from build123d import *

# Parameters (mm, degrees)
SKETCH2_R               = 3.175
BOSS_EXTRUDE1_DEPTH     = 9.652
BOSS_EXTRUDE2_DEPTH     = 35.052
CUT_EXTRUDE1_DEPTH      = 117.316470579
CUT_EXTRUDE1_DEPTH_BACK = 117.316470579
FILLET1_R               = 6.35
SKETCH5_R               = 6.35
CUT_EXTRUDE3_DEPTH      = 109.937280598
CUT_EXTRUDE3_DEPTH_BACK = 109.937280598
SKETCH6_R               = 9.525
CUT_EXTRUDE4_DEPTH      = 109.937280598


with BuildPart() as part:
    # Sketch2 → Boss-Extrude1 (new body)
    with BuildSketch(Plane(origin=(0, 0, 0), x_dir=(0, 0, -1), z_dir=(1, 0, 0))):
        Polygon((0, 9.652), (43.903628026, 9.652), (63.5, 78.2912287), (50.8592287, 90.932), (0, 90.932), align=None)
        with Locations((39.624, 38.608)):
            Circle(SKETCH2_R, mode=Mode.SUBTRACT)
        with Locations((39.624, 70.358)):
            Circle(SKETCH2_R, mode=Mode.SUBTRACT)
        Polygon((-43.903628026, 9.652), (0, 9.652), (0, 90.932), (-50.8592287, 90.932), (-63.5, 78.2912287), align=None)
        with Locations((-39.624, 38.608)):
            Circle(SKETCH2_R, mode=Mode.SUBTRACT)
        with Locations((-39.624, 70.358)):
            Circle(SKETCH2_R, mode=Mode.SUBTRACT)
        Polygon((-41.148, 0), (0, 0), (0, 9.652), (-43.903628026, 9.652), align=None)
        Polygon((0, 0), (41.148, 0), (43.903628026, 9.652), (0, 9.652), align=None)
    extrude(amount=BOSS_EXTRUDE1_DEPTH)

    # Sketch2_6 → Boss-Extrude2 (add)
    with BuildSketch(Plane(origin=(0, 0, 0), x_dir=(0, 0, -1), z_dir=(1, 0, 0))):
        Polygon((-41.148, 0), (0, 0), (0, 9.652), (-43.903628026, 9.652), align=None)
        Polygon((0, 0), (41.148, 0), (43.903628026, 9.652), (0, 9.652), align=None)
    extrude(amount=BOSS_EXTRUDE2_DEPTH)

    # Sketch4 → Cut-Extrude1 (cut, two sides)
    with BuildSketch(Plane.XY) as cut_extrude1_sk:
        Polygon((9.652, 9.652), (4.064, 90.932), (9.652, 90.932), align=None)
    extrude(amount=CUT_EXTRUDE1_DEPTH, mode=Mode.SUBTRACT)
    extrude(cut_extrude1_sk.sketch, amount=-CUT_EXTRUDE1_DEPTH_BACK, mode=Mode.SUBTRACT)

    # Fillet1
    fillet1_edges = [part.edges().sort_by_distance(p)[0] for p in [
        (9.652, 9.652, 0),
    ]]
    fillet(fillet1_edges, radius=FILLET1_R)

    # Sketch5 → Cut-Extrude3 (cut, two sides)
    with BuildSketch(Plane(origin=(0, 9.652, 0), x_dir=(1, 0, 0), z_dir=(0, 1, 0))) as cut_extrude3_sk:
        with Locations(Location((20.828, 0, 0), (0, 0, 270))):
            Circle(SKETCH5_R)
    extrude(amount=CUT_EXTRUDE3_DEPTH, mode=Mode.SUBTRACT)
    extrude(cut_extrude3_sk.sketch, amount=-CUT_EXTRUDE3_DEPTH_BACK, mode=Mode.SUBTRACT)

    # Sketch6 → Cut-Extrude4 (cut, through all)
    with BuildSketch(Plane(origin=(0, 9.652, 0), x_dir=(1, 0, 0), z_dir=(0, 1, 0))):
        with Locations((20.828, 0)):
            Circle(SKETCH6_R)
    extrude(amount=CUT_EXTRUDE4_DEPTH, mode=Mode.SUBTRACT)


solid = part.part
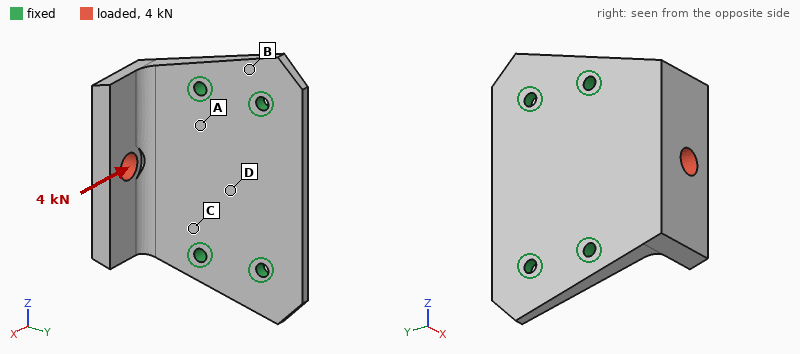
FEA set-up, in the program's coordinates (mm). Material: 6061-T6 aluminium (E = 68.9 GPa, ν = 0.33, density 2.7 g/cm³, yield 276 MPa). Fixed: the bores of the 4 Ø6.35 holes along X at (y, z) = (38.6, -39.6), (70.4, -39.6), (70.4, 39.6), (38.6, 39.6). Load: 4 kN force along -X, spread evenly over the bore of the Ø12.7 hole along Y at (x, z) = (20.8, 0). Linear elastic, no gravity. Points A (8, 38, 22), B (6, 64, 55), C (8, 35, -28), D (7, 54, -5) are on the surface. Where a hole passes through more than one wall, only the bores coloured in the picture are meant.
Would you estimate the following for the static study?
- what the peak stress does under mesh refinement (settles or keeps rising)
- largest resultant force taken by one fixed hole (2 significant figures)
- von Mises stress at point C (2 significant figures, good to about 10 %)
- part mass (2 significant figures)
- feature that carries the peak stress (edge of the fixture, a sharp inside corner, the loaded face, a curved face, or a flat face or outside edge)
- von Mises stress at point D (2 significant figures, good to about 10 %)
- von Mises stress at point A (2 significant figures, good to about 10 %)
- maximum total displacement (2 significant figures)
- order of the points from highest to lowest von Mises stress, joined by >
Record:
keeps rising
2.7 kN
85 MPa
230 g
edge of the fixture
30 MPa
67 MPa
0.40 mm
C > A > D > B
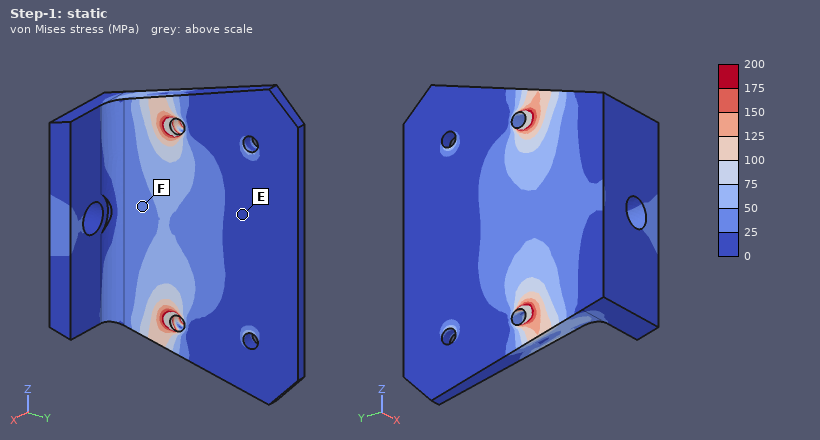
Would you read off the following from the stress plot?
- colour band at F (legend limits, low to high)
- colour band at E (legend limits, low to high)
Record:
25 to 50 MPa
0 to 25 MPa
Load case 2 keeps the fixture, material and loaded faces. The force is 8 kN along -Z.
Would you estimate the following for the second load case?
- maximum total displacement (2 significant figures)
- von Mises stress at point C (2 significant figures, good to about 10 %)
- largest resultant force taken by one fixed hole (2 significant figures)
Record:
0.14 mm
42 MPa
5.0 kN
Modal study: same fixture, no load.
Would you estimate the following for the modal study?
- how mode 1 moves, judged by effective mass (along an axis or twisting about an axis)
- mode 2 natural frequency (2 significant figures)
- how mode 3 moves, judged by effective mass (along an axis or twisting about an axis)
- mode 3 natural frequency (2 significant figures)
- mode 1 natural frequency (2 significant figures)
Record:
along X
4000 Hz
along X
4600 Hz
1900 Hz
